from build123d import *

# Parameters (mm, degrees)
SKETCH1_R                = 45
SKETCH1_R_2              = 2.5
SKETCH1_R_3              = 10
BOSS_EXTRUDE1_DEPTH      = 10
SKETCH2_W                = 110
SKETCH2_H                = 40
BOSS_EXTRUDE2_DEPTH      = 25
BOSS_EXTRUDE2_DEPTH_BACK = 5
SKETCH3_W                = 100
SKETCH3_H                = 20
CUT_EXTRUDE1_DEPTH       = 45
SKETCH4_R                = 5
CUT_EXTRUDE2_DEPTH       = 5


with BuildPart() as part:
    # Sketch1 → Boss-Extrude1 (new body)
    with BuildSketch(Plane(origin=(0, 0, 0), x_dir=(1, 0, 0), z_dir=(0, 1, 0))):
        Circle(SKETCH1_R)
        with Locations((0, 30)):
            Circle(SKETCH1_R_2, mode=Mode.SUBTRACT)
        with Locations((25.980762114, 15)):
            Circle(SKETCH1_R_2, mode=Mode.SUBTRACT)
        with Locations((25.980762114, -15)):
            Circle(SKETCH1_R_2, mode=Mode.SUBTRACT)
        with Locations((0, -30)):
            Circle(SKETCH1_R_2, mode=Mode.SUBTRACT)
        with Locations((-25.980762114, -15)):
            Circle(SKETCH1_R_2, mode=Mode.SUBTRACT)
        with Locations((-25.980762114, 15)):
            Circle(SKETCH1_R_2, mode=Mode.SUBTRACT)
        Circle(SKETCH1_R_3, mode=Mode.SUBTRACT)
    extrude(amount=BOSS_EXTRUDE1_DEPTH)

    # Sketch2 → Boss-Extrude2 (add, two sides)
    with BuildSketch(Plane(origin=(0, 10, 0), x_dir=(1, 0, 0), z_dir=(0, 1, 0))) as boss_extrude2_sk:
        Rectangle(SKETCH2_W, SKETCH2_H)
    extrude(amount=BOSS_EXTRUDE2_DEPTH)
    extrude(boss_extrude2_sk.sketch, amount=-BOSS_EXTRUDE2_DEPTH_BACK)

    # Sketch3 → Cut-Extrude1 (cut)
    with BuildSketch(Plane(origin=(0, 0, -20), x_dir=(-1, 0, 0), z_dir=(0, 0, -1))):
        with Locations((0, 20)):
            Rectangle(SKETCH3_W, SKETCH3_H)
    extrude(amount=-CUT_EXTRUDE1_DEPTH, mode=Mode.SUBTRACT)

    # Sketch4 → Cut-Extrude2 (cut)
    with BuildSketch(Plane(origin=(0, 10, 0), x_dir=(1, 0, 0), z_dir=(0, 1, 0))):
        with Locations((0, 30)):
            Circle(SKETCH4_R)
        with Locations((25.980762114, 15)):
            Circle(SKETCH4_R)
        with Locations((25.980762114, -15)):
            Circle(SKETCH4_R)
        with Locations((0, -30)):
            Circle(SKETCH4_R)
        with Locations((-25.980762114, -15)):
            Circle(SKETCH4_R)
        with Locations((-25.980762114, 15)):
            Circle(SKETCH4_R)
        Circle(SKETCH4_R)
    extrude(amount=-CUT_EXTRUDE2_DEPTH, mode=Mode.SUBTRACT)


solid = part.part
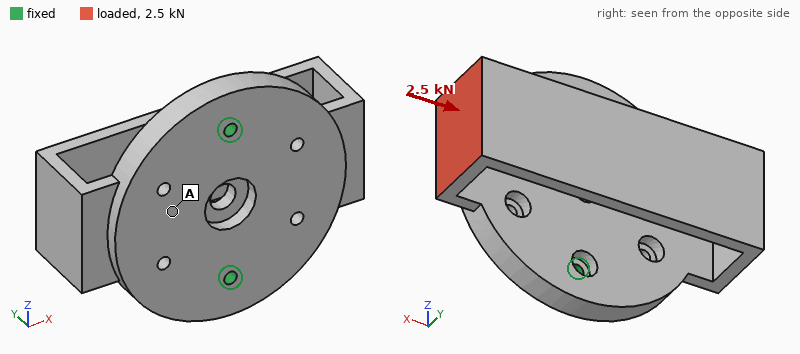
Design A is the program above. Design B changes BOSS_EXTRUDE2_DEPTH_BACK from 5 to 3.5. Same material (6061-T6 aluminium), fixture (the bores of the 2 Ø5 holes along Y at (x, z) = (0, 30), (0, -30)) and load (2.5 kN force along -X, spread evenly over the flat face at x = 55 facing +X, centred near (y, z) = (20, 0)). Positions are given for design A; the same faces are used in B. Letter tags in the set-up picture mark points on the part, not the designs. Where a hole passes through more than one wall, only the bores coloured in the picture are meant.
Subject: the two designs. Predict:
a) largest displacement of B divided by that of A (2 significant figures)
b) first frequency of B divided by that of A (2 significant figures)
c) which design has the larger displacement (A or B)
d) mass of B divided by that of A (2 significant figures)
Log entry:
1.2
0.99
B
0.98
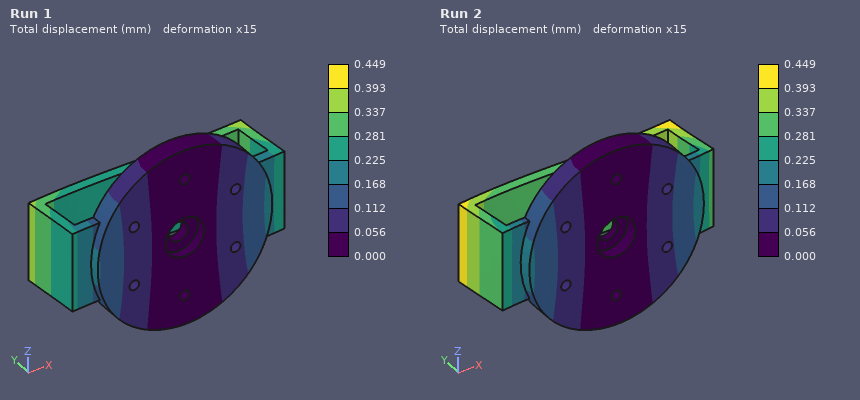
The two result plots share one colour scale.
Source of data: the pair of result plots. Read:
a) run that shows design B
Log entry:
Run 2
